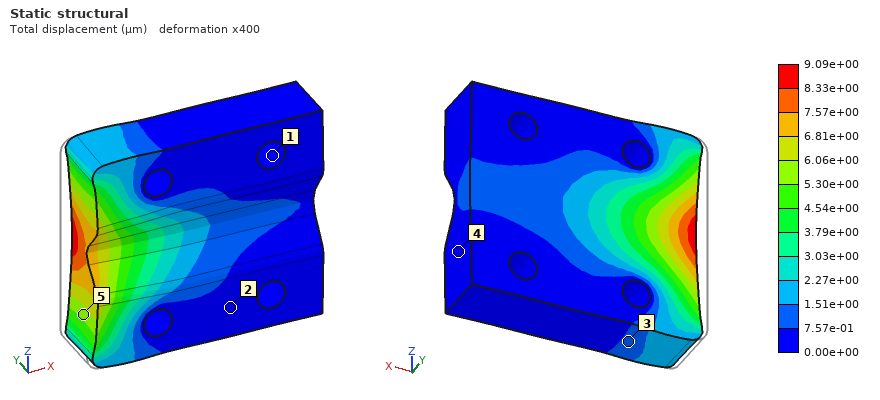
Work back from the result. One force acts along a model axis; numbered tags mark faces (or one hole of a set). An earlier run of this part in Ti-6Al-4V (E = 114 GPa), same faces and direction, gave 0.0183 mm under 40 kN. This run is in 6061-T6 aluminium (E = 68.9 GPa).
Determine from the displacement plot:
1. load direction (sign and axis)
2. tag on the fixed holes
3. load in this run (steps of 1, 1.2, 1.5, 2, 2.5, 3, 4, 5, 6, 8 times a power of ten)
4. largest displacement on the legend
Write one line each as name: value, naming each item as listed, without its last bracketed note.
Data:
load direction: +X
tag on the fixed holes: 1
load in this run: 12 kN
largest displacement on the legend: 9.09e+00 µm
